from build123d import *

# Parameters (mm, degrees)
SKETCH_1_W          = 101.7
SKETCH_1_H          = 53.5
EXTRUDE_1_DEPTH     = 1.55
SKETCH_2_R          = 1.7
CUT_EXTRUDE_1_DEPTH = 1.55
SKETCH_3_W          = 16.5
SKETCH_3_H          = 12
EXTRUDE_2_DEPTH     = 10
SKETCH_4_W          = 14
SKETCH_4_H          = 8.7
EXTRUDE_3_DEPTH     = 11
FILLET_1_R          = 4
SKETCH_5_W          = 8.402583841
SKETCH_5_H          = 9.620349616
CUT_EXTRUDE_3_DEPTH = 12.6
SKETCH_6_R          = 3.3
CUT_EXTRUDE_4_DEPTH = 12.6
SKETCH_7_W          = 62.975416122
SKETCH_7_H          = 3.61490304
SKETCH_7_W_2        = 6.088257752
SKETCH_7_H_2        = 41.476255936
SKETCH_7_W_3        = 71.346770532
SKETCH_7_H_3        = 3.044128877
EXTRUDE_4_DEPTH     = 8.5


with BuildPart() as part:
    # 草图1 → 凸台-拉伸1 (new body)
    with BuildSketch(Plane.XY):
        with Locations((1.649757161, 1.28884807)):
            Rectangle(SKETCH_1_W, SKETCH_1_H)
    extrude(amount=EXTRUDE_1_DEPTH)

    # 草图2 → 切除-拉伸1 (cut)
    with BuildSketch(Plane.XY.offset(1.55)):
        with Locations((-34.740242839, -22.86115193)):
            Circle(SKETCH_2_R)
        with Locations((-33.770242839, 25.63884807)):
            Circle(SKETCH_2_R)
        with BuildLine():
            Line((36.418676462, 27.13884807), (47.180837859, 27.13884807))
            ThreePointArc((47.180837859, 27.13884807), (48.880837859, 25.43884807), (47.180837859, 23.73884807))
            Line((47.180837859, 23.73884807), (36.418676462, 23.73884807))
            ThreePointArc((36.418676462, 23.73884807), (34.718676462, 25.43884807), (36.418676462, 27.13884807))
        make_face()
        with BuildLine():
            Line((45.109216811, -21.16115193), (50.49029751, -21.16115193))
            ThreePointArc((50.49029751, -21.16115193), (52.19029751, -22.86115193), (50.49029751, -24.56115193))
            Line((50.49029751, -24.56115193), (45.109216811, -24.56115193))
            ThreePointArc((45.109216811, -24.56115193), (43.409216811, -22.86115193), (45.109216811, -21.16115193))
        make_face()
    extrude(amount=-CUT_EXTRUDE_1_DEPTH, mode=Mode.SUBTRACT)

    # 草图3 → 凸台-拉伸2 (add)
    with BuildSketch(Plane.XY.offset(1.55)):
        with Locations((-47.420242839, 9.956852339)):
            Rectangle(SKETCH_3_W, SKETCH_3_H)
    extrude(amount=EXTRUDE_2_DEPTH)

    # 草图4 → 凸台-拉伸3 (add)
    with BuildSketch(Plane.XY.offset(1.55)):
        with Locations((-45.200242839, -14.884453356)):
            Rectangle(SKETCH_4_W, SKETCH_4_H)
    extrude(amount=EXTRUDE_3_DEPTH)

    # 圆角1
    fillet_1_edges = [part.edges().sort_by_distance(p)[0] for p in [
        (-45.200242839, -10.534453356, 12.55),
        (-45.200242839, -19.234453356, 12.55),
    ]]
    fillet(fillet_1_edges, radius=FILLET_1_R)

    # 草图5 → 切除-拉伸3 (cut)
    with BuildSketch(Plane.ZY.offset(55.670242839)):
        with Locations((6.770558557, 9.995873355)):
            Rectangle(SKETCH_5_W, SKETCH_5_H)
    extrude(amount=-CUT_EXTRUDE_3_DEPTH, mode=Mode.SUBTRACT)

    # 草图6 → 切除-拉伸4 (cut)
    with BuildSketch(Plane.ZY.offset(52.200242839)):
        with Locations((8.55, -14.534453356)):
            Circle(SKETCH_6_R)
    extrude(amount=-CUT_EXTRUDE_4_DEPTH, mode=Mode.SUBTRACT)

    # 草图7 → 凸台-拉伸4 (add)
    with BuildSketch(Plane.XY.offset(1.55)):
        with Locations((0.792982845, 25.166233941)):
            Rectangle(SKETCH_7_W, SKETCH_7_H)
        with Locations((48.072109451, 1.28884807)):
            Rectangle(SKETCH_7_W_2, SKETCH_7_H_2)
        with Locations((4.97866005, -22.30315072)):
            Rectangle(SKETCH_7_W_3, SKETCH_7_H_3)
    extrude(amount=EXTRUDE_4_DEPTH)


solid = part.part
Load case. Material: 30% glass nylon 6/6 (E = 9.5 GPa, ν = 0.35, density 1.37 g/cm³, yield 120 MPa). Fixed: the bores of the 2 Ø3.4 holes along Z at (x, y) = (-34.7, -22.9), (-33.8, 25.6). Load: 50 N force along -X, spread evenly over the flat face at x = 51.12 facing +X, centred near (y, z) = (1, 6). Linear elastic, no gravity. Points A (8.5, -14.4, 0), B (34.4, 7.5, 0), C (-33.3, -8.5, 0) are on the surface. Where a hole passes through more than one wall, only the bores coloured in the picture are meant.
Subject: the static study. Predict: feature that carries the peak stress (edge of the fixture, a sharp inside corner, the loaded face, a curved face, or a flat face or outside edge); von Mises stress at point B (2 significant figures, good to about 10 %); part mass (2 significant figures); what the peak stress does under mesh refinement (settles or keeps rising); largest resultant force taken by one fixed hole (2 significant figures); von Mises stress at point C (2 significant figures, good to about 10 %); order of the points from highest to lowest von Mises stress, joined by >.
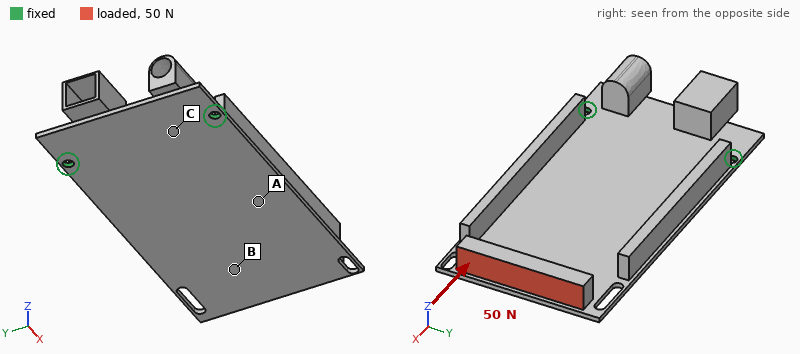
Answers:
edge of the fixture
6.4 MPa
22 g
keeps rising
25 N
3.6 MPa
B > C > A
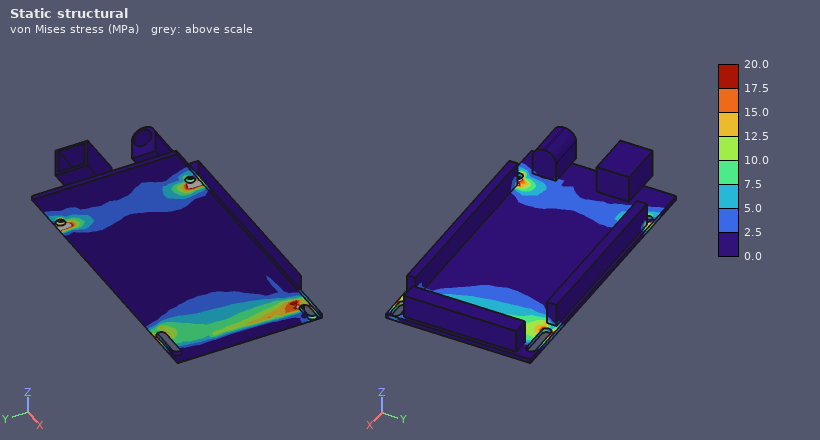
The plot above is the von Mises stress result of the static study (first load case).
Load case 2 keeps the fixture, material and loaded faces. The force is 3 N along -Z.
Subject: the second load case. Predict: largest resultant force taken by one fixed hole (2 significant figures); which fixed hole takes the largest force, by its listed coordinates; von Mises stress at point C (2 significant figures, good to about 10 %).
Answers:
1.9 N
(-33.8, 25.6)
3.7 MPa
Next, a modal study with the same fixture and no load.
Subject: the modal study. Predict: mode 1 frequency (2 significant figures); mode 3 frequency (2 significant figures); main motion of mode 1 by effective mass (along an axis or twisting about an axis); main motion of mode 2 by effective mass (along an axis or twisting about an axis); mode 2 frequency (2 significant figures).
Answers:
97 Hz
890 Hz
along Z
twisting about X
330 Hz
